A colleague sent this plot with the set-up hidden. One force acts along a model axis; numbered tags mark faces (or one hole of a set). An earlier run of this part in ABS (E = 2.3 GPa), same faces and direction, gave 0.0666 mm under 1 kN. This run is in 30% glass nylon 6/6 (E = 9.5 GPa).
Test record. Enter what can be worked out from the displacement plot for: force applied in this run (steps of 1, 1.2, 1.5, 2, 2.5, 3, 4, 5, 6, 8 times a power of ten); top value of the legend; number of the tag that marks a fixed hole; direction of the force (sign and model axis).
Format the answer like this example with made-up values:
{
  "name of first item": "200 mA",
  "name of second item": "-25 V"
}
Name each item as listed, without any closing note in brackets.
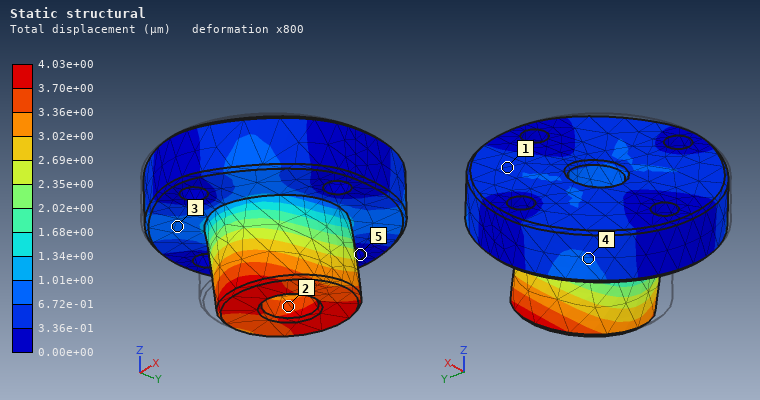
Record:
{
  "force applied in this run": "250 N",
  "top value of the legend": "4.03e+00 µm",
  "number of the tag that marks a fixed hole": "5",
  "direction of the force": "+Y"
}
